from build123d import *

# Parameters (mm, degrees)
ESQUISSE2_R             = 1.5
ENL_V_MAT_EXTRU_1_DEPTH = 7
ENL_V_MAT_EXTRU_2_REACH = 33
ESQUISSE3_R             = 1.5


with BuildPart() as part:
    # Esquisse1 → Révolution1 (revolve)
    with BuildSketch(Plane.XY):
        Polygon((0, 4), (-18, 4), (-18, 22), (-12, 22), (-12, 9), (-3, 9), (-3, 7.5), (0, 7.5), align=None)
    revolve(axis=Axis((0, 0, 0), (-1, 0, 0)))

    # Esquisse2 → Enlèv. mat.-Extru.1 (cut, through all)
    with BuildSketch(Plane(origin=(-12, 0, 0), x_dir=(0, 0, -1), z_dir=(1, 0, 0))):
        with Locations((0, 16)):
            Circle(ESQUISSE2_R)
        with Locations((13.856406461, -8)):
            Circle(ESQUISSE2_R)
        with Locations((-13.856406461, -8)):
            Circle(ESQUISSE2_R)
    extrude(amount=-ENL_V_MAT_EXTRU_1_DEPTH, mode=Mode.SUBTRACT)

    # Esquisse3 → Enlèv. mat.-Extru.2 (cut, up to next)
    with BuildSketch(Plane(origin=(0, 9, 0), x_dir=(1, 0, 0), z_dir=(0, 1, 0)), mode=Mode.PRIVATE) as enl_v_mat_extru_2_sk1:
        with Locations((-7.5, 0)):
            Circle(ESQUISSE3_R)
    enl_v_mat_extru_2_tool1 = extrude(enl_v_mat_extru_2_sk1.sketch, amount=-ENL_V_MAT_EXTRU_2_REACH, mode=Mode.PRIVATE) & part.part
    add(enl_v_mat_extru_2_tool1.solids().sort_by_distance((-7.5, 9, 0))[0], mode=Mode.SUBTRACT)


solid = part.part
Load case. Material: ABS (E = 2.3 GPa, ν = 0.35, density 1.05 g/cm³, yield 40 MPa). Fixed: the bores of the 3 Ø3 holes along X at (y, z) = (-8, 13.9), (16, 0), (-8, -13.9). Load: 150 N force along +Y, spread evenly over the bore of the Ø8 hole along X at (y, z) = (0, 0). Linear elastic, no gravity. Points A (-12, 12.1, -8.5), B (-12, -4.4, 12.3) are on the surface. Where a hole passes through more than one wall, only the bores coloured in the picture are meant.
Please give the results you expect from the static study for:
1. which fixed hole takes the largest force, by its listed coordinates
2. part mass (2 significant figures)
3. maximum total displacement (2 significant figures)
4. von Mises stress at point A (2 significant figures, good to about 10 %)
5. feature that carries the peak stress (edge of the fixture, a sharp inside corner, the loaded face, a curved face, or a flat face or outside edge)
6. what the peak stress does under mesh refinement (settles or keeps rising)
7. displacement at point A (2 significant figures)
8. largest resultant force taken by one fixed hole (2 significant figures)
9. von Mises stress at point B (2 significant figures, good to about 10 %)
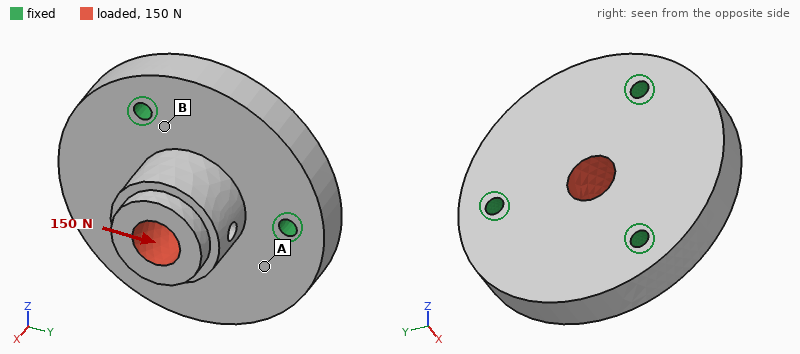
(16, 0)
11 g
25 µm
0.46 MPa
edge of the fixture
keeps rising
4.7 µm
67 N
1.2 MPa
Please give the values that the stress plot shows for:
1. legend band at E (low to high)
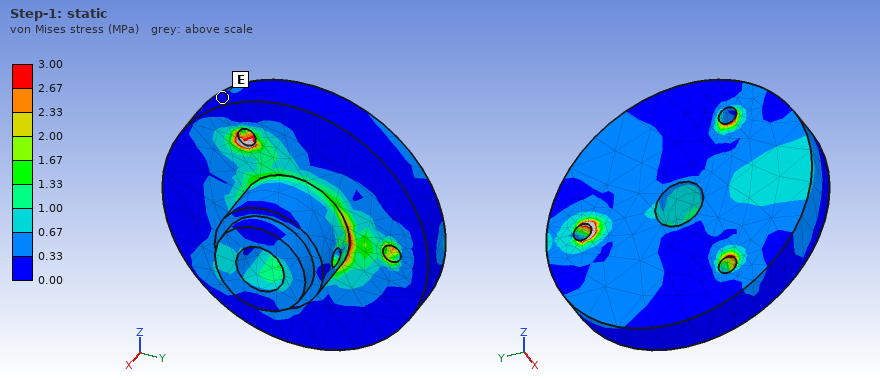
0.00 to 0.33 MPa
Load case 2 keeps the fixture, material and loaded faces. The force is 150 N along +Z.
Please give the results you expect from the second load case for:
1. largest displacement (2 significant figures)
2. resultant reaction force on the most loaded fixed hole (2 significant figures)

25 µm
62 N
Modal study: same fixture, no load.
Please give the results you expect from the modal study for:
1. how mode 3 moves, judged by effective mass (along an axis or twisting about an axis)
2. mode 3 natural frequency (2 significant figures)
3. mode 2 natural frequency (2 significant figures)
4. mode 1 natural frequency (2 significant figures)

along X
6200 Hz
5500 Hz
5500 Hz
